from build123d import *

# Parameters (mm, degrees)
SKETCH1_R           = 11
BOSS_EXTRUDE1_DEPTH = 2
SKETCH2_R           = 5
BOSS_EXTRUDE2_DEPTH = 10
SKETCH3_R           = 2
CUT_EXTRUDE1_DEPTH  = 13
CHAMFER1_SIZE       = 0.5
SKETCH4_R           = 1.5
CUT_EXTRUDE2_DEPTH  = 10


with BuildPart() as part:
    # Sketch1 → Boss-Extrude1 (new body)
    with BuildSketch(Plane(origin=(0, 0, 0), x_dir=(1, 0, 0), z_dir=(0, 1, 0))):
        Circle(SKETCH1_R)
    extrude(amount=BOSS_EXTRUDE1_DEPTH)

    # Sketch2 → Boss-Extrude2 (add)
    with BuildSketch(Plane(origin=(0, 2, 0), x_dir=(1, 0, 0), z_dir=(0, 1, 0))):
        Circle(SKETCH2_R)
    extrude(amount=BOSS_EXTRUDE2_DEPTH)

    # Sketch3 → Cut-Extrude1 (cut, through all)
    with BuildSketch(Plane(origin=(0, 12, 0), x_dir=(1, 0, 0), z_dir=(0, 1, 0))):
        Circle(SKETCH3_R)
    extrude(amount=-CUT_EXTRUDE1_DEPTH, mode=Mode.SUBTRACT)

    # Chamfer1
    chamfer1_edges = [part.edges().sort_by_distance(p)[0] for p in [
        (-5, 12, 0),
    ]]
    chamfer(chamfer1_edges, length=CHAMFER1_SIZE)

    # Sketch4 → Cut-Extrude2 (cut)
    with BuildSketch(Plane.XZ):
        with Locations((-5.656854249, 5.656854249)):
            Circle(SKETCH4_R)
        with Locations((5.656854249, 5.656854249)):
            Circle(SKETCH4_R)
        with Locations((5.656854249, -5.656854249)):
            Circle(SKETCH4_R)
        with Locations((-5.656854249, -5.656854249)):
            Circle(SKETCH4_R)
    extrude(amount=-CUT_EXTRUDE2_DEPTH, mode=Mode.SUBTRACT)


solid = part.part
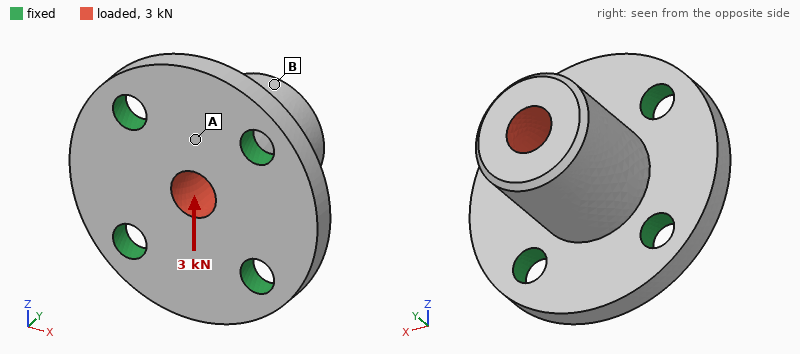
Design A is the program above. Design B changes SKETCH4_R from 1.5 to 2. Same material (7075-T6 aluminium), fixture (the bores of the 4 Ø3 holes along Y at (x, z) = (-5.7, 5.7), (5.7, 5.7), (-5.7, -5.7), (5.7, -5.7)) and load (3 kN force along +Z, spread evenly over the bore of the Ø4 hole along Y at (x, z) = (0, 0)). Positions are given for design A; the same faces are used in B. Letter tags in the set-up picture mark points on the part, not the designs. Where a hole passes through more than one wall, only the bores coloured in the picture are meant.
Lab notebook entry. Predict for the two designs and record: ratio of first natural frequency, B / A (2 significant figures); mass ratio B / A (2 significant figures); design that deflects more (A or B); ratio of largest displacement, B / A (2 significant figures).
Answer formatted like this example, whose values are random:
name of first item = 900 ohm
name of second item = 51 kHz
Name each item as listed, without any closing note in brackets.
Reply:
ratio of first natural frequency, B / A = 1.1
mass ratio B / A = 0.97
design that deflects more = A
ratio of largest displacement, B / A = 0.83
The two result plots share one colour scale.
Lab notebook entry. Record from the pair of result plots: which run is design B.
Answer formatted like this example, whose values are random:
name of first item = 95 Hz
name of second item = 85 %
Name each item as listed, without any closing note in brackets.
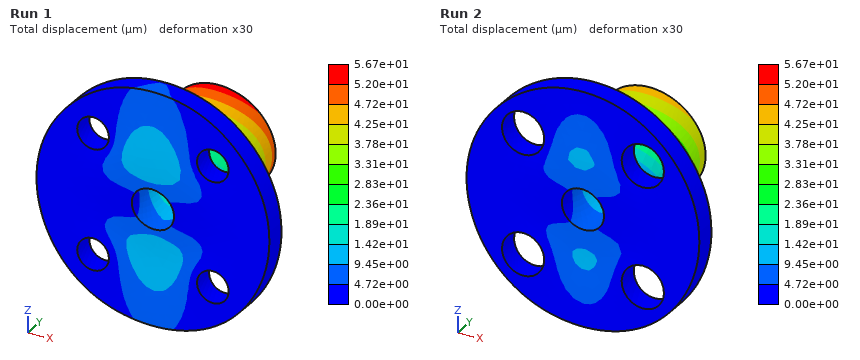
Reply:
which run is design B = Run 2
